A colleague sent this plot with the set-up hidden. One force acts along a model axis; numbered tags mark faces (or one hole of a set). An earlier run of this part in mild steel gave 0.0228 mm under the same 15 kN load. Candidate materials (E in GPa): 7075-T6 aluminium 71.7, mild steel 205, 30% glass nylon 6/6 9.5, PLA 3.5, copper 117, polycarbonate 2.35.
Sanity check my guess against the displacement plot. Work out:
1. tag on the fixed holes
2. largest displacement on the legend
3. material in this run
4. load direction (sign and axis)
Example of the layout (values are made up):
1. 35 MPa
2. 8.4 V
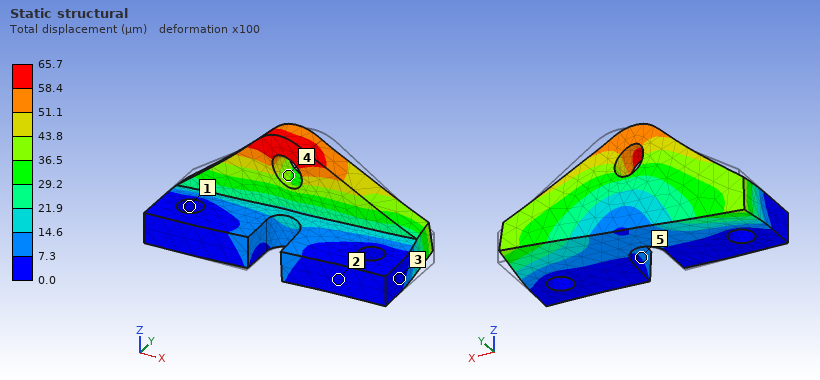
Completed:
1. 1
2. 65.7 µm
3. 7075-T6 aluminium
4. -X
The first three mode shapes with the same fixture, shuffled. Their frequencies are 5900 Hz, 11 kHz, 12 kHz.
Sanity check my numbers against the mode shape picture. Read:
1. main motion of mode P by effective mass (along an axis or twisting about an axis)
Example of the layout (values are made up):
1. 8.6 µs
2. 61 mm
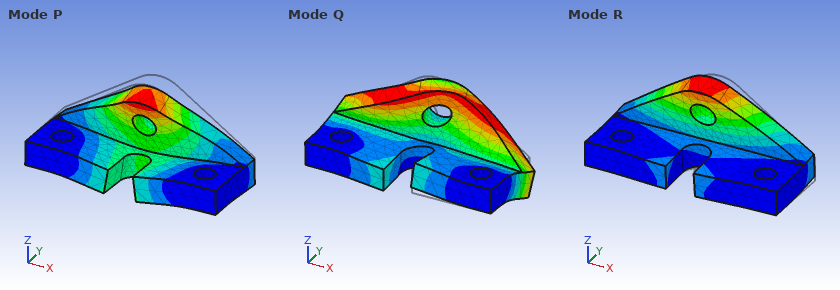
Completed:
1. along Z
